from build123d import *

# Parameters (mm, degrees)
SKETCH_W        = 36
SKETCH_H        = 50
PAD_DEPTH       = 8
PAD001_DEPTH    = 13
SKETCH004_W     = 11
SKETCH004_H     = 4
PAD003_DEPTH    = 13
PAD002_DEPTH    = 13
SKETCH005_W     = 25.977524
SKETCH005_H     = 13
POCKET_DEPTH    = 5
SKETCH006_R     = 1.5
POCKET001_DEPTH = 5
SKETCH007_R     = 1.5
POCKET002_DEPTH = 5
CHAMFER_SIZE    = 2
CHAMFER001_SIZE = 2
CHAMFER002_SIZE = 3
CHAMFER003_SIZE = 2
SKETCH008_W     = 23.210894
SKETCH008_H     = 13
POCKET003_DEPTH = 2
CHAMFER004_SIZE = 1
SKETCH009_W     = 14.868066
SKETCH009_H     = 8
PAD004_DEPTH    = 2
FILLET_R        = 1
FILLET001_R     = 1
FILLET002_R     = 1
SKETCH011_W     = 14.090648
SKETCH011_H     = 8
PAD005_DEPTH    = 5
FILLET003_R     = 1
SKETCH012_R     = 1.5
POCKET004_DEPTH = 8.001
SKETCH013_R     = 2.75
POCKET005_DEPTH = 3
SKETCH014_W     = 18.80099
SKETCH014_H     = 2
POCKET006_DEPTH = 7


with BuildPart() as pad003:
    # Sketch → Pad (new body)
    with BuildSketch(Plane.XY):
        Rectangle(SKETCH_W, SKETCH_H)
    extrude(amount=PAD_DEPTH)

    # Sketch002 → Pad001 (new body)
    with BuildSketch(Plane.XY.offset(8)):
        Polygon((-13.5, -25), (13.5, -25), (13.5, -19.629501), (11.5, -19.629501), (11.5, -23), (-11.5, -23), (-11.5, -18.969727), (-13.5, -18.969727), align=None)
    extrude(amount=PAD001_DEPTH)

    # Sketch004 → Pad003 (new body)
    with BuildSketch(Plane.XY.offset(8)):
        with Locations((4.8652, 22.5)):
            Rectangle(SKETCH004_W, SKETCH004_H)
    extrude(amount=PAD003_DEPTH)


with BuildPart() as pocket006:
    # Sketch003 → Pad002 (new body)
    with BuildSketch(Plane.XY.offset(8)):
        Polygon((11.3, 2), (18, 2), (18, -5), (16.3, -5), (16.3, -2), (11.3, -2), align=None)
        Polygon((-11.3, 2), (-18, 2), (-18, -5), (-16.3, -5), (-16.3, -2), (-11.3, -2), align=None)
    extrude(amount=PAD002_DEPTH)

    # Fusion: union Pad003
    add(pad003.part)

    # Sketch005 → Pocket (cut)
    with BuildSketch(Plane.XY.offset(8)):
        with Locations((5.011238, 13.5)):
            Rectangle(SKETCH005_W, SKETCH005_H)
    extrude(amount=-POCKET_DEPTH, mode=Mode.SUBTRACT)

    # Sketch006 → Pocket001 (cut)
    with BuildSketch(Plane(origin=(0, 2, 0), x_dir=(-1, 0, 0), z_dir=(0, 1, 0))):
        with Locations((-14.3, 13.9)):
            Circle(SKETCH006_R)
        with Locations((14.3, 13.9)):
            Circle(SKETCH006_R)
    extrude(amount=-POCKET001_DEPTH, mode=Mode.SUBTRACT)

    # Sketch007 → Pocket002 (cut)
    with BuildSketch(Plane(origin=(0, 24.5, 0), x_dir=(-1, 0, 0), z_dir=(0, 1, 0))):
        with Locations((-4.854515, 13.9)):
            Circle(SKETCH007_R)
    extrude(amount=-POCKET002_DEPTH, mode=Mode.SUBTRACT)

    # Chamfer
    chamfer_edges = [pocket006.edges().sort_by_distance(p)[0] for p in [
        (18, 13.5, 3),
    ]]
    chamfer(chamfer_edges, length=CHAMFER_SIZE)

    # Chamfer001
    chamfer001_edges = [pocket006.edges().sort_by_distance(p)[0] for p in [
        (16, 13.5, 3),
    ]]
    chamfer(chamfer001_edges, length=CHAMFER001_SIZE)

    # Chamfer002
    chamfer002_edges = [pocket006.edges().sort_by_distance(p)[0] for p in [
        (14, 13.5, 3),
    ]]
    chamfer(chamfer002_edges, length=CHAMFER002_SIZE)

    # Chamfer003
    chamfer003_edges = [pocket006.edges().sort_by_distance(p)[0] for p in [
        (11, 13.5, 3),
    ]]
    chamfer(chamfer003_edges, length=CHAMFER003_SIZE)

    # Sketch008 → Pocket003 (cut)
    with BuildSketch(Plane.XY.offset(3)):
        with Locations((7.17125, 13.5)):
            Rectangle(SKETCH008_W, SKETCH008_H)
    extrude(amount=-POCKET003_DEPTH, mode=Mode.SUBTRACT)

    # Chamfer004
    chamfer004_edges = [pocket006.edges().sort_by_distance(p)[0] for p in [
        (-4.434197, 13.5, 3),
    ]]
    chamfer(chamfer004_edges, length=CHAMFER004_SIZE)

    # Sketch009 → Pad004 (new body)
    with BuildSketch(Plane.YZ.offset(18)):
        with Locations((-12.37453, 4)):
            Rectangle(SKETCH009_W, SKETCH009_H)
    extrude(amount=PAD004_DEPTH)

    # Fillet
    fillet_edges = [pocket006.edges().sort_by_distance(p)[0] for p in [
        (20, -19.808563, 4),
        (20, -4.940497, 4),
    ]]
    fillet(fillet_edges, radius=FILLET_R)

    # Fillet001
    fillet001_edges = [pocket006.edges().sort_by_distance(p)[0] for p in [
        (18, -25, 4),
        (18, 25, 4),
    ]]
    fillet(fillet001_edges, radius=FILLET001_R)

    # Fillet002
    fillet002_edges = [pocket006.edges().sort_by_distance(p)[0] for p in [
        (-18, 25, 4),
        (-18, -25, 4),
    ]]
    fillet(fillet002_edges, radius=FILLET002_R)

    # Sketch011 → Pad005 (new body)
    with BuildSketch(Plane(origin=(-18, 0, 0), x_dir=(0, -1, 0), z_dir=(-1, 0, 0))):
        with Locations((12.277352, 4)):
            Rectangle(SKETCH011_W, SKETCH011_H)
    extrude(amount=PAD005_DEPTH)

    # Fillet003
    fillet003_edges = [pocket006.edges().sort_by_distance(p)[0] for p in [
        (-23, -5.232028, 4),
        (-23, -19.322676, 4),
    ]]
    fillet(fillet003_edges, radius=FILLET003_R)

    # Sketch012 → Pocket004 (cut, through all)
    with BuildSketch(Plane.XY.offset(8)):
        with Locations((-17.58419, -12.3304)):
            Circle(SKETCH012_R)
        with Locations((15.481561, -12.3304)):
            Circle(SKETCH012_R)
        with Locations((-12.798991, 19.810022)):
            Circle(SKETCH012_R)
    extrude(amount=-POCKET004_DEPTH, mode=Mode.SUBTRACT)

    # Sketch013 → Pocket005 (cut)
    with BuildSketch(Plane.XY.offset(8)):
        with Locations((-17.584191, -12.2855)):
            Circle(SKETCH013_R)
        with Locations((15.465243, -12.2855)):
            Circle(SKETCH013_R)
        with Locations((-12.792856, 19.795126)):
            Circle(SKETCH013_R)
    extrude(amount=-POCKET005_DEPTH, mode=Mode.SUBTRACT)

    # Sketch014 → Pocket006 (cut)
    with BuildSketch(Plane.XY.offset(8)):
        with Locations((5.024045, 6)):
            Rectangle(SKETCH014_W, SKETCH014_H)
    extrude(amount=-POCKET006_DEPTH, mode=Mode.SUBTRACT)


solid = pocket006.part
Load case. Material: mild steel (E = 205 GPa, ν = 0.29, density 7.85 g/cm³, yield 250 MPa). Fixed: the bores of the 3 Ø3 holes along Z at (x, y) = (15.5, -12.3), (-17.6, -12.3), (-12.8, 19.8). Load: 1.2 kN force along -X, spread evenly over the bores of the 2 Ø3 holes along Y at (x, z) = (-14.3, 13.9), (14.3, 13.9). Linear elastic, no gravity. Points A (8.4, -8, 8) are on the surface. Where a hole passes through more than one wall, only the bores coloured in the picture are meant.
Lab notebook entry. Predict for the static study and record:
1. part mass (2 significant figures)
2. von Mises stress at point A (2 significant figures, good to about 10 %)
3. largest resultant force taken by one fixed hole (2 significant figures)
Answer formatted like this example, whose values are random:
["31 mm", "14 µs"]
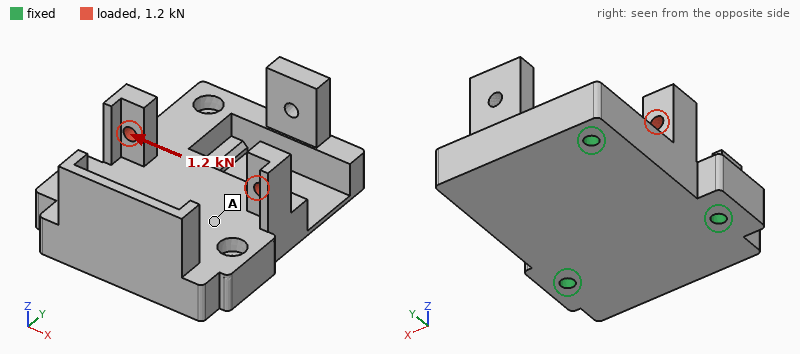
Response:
["110 g", "17 MPa", "740 N"]
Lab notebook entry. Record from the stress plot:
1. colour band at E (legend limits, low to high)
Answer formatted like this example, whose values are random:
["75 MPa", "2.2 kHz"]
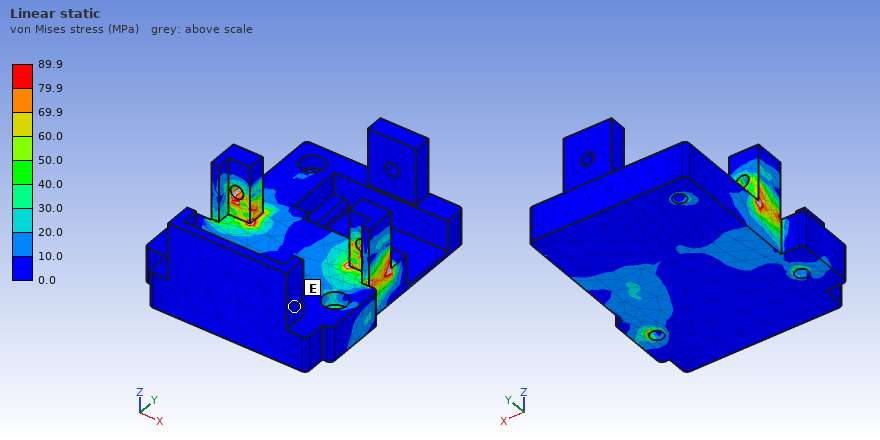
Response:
["0.0 to 10.0 MPa"]
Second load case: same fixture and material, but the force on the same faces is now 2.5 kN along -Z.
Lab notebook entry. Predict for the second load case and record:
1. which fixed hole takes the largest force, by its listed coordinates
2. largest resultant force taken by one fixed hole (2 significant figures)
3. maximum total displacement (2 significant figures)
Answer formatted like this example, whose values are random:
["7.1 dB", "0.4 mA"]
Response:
["(15.5, -12.3)", "1.2 kN", "27 µm"]
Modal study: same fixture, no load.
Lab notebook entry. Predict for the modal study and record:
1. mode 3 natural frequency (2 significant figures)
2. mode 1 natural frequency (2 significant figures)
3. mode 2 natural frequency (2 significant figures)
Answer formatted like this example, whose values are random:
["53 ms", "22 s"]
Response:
["9600 Hz", "5100 Hz", "6100 Hz"]
